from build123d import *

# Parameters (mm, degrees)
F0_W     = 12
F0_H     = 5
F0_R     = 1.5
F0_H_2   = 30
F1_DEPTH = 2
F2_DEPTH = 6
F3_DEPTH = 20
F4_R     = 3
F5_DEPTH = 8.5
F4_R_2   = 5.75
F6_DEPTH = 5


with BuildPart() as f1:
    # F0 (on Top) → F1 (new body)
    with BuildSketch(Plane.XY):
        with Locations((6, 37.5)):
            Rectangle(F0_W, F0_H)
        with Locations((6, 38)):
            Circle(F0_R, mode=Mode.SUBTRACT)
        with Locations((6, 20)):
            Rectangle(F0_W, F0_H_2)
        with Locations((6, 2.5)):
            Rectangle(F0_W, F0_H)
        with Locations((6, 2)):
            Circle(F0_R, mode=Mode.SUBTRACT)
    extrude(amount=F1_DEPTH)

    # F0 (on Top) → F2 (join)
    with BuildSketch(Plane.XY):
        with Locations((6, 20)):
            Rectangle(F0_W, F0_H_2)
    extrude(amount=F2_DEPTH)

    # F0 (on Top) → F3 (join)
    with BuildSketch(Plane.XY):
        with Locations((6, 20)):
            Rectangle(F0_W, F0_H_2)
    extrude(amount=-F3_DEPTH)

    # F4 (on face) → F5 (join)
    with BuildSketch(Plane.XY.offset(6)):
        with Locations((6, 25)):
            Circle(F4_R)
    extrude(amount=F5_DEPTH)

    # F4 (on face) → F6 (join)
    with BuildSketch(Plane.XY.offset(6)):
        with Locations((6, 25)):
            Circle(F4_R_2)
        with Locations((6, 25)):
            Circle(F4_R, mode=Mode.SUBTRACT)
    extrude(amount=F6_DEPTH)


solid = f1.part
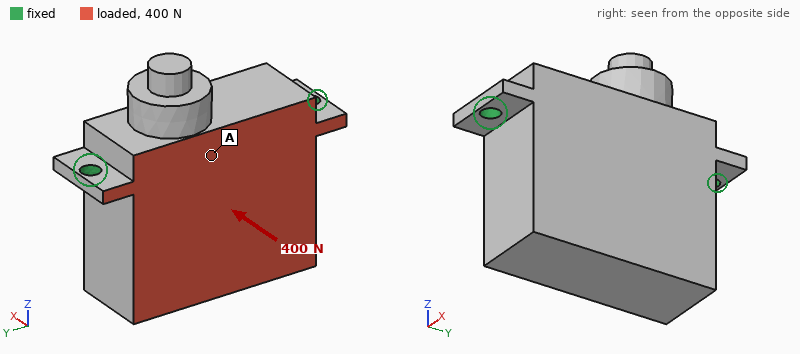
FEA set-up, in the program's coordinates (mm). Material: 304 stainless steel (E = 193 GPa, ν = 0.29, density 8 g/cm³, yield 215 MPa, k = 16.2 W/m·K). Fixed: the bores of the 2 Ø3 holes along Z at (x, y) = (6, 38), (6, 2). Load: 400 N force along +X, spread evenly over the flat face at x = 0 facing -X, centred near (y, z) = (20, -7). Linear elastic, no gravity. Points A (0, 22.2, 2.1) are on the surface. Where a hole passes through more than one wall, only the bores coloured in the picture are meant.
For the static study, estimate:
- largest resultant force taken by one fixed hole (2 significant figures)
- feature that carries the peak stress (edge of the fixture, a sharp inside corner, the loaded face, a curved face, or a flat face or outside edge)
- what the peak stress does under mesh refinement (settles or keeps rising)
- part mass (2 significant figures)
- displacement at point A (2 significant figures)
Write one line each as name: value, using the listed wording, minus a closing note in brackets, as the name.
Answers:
largest resultant force taken by one fixed hole: 200 N
feature that carries the peak stress: edge of the fixture
what the peak stress does under mesh refinement: keeps rising
part mass: 82 g
displacement at point A: 8.3 µm
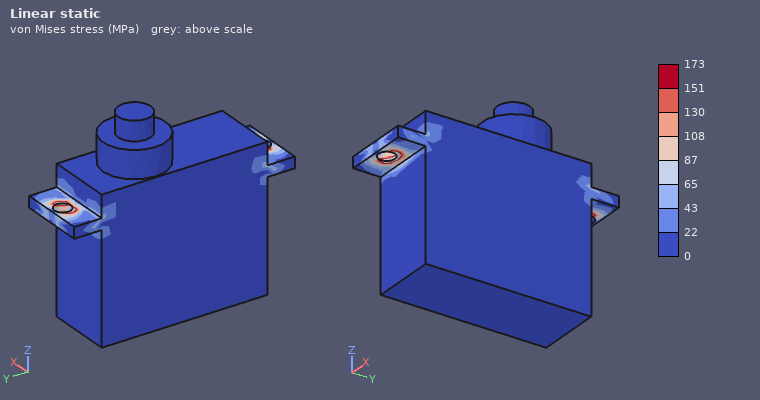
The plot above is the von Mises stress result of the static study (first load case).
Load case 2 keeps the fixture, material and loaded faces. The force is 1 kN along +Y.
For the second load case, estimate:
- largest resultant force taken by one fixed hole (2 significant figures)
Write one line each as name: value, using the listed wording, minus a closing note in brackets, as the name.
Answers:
largest resultant force taken by one fixed hole: 580 N
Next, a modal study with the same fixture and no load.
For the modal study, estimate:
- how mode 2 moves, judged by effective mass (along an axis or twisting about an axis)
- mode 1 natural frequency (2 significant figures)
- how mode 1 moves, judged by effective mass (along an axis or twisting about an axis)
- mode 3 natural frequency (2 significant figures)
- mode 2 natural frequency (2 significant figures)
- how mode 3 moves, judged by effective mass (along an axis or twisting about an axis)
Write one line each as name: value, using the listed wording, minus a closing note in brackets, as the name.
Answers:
how mode 2 moves, judged by effective mass: along Z
mode 1 natural frequency: 2300 Hz
how mode 1 moves, judged by effective mass: along X
mode 3 natural frequency: 12 kHz
mode 2 natural frequency: 11 kHz
how mode 3 moves, judged by effective mass: along Y
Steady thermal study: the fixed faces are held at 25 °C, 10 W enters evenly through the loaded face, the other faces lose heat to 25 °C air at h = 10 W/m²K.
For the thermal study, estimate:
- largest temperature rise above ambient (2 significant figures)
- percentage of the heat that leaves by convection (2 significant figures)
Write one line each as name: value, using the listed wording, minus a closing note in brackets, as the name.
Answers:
largest temperature rise above ambient: 68 K
percentage of the heat that leaves by convection: 14 %
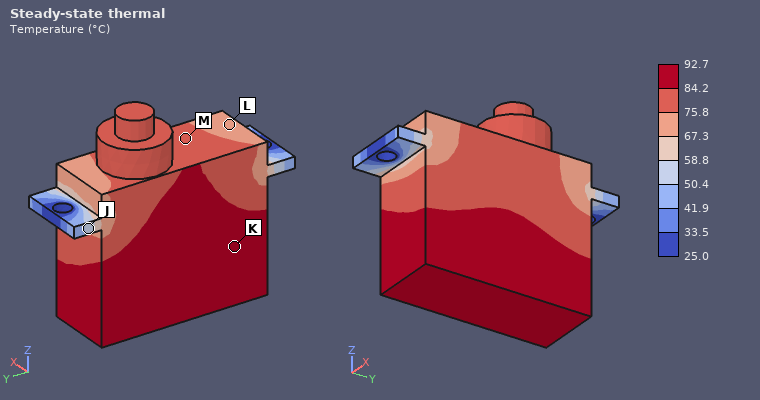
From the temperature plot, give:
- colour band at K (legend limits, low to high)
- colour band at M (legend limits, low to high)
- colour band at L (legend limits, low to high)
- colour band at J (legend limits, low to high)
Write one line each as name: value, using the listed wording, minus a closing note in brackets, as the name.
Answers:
colour band at K: 84.2 to 92.7 °C
colour band at M: 75.8 to 84.2 °C
colour band at L: 67.3 to 75.8 °C
colour band at J: 50.4 to 58.8 °C
